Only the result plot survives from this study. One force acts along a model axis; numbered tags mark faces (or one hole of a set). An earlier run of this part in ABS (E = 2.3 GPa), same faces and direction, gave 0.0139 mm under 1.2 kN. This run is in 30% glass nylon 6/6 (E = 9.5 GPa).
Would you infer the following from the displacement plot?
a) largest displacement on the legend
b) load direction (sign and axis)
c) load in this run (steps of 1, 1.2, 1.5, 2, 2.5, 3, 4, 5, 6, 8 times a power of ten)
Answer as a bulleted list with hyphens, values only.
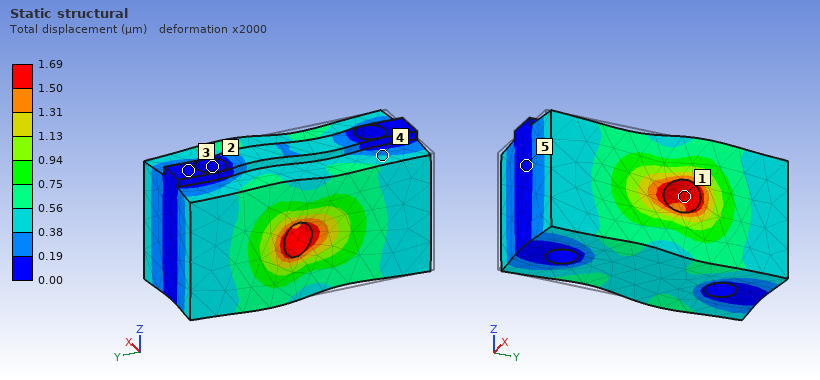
- 1.69 µm
- +Y
- 600 N
